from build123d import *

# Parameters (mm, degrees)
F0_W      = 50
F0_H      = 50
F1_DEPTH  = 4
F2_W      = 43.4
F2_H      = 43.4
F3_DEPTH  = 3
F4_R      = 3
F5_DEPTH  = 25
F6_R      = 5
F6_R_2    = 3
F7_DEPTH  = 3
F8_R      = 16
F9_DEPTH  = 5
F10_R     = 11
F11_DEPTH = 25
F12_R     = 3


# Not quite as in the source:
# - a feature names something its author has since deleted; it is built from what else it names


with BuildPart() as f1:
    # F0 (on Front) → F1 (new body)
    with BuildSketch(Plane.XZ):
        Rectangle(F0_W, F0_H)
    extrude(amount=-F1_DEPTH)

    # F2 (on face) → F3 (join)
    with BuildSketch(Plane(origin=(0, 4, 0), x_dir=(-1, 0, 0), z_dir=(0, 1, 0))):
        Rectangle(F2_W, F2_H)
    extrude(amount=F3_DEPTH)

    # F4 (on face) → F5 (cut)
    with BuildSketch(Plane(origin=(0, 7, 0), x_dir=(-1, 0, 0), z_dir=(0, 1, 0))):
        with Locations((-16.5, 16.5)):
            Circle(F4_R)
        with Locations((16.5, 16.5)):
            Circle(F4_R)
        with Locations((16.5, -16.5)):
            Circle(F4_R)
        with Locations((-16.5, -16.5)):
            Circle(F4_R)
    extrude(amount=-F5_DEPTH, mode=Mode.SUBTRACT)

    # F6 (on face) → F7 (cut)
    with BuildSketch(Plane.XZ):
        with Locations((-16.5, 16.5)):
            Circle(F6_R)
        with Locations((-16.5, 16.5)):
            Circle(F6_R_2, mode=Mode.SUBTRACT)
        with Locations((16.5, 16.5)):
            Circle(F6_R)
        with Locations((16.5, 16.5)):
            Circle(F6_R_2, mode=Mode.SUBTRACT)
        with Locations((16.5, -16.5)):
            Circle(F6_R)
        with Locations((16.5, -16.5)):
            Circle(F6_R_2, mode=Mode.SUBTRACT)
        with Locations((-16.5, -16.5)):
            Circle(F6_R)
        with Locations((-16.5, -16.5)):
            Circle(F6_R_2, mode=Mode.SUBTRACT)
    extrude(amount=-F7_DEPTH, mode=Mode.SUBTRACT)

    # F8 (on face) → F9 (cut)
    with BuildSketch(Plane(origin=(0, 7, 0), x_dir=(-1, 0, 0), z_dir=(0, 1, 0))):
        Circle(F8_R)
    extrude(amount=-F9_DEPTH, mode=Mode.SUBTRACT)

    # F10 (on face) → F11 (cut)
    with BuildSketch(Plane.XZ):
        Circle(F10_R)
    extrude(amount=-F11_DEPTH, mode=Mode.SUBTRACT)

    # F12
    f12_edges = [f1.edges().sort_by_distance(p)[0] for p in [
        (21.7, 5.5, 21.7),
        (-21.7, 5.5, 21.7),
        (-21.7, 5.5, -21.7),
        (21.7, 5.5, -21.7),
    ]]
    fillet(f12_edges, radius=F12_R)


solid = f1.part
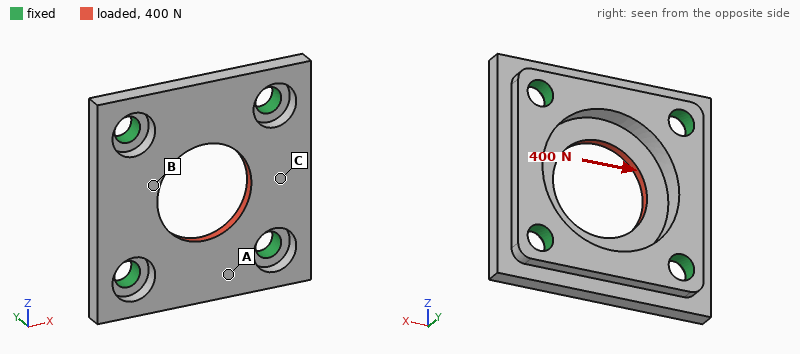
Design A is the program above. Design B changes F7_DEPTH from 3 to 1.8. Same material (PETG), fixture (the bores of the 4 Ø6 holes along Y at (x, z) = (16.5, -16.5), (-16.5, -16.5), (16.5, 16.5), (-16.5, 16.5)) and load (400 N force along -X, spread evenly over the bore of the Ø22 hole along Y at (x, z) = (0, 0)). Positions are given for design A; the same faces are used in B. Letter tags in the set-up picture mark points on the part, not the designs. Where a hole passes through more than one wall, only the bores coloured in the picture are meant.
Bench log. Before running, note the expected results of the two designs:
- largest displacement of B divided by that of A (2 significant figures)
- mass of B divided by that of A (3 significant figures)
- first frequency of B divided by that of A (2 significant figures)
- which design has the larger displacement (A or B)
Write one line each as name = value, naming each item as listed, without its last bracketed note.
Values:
largest displacement of B divided by that of A = 0.84
mass of B divided by that of A = 1.03
first frequency of B divided by that of A = 1.1
which design has the larger displacement = A
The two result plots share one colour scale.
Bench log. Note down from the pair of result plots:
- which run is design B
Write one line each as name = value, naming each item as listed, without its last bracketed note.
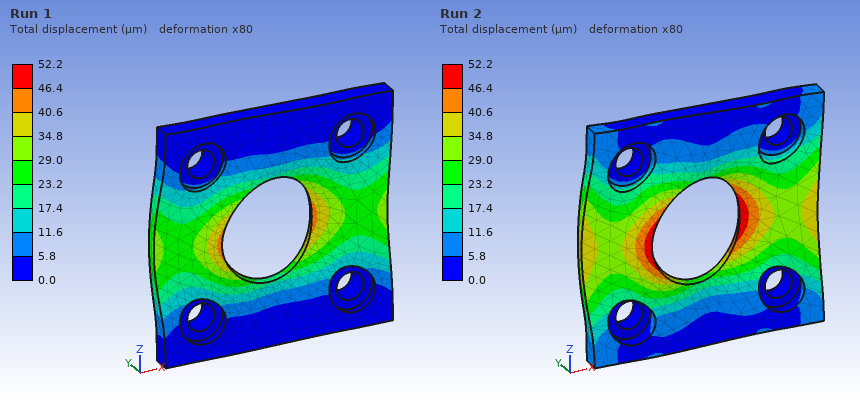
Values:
which run is design B = Run 1
